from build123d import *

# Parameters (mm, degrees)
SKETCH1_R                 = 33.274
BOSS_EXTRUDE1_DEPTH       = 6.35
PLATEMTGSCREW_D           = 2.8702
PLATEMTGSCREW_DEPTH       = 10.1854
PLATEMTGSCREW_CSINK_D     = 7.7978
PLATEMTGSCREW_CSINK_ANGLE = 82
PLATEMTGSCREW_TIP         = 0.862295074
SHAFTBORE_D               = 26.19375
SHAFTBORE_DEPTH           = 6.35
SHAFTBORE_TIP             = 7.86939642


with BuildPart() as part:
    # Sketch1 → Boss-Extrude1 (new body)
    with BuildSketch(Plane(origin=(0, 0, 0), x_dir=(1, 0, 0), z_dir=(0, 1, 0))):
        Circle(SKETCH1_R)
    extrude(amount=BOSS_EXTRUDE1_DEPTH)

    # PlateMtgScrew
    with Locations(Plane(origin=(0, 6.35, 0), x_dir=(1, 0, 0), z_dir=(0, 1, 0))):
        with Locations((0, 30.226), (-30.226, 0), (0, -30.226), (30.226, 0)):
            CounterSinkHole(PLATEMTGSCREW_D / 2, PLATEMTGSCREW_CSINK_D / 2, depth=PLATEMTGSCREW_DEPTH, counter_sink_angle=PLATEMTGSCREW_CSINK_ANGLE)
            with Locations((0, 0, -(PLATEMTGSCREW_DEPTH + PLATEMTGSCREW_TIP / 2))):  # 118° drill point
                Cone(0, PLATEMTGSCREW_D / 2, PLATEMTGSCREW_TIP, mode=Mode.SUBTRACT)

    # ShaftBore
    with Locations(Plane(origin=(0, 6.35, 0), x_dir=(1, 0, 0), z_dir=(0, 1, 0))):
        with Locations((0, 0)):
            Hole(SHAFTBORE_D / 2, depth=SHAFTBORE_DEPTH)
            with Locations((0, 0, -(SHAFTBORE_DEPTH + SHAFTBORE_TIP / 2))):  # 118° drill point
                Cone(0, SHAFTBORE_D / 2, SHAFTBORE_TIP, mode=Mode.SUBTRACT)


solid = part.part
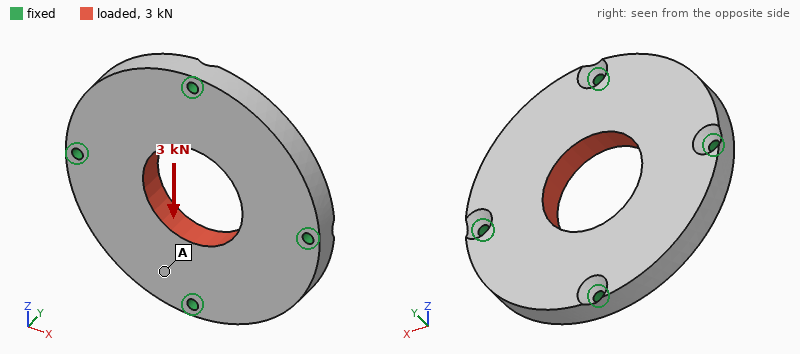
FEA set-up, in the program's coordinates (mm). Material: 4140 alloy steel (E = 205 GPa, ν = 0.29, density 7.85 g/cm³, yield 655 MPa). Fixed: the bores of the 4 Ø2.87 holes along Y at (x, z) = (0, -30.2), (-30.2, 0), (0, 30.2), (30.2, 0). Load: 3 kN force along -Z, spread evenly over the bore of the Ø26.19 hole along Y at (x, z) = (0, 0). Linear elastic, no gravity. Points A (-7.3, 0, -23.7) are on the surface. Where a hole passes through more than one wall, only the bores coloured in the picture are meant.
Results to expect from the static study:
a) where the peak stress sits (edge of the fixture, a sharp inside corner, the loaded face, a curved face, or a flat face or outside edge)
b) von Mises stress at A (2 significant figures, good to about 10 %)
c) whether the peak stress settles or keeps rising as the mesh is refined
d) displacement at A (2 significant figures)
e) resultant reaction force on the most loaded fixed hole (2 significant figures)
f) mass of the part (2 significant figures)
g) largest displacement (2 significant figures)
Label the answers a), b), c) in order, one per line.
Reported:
a) edge of the fixture
b) 7.8 MPa
c) keeps rising
d) 0.78 µm
e) 840 N
f) 140 g
g) 1.4 µm
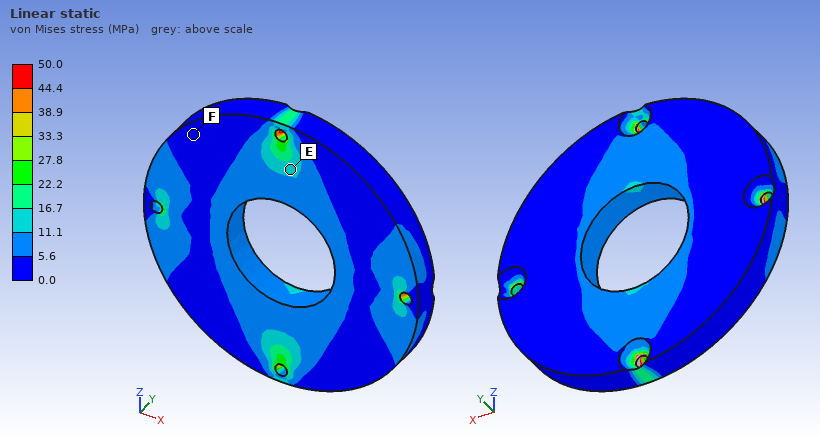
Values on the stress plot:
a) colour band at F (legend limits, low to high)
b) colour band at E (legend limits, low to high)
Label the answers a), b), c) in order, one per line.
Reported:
a) 0.0 to 5.6 MPa
b) 11.1 to 16.7 MPa
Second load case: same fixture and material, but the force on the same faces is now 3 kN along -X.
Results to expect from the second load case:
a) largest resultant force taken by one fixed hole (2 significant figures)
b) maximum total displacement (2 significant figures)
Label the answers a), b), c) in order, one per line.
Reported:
a) 840 N
b) 1.4 µm
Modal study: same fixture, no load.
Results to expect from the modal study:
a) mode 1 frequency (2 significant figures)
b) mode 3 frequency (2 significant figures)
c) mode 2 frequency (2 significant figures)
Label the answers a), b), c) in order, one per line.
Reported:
a) 9900 Hz
b) 11 kHz
c) 10 kHz
